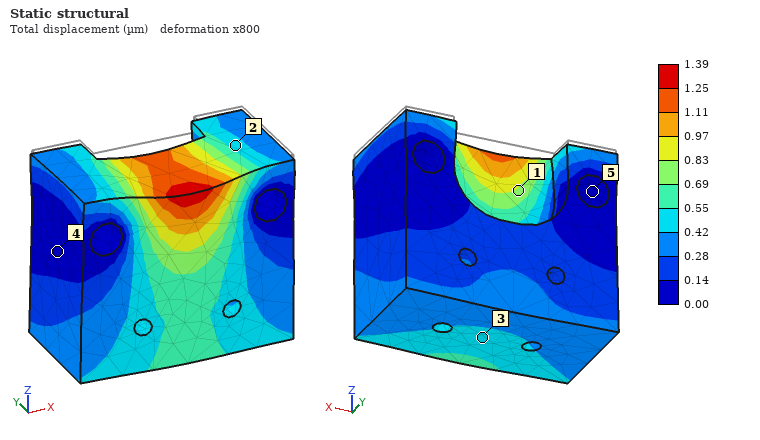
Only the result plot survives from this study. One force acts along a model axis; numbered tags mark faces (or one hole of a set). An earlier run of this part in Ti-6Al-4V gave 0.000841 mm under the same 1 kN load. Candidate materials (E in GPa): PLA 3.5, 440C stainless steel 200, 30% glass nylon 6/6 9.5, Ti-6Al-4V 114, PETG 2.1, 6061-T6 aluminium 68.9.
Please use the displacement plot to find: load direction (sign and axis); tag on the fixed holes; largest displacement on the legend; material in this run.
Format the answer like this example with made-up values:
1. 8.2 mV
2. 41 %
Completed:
1. -Z
2. 5
3. 1.39 µm
4. 6061-T6 aluminium
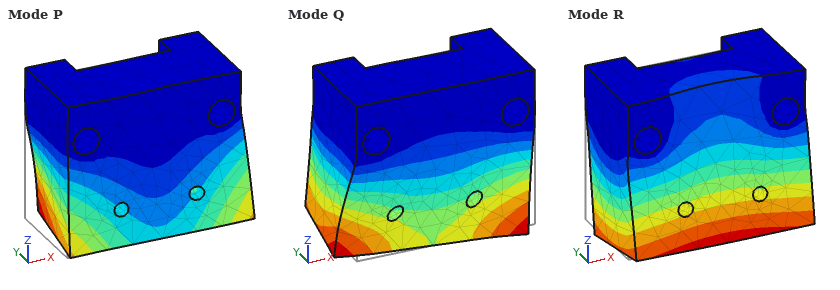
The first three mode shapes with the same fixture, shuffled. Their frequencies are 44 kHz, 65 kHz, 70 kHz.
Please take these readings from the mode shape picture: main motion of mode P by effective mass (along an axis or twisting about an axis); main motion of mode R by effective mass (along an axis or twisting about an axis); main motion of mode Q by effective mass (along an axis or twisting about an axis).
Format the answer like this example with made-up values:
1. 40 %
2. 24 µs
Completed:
1. along X
2. along Y
3. along X
